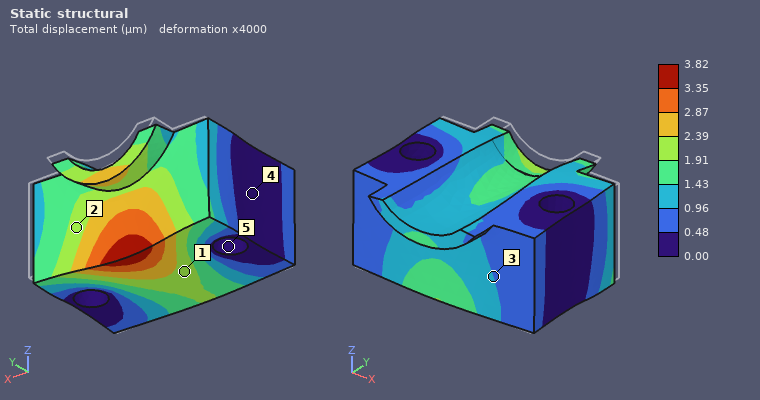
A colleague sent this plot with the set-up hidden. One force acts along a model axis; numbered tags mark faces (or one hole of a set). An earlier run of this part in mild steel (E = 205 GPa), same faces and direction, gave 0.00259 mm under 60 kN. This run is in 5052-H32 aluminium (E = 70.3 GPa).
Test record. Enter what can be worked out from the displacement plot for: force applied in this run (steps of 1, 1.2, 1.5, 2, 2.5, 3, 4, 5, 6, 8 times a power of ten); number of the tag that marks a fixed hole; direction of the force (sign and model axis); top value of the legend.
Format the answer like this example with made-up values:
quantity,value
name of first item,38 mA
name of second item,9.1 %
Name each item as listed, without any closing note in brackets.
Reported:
quantity,value
force applied in this run,30 kN
number of the tag that marks a fixed hole,5
direction of the force,-Y
top value of the legend,3.82 µm
